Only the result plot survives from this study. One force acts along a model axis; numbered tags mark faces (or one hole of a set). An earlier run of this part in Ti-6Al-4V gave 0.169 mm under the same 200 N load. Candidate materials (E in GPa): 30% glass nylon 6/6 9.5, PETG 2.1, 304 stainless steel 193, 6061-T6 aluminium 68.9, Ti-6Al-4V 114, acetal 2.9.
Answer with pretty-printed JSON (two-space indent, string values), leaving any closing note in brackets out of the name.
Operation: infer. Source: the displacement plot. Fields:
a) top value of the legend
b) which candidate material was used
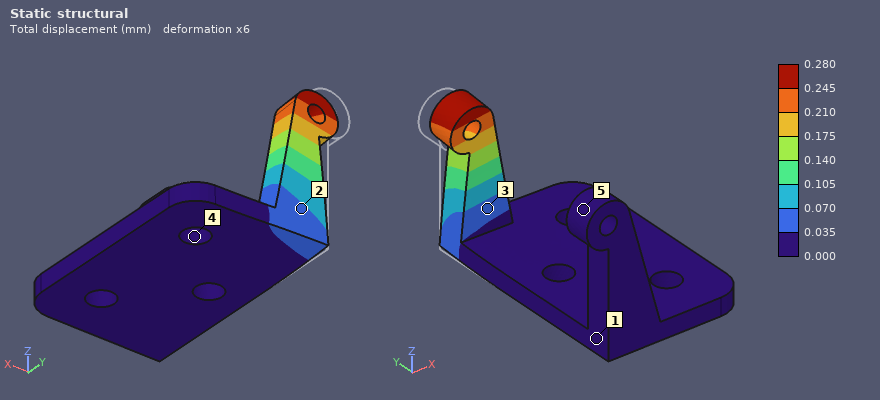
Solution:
{
  "top value of the legend": "0.280 mm",
  "which candidate material was used": "6061-T6 aluminium"
}
